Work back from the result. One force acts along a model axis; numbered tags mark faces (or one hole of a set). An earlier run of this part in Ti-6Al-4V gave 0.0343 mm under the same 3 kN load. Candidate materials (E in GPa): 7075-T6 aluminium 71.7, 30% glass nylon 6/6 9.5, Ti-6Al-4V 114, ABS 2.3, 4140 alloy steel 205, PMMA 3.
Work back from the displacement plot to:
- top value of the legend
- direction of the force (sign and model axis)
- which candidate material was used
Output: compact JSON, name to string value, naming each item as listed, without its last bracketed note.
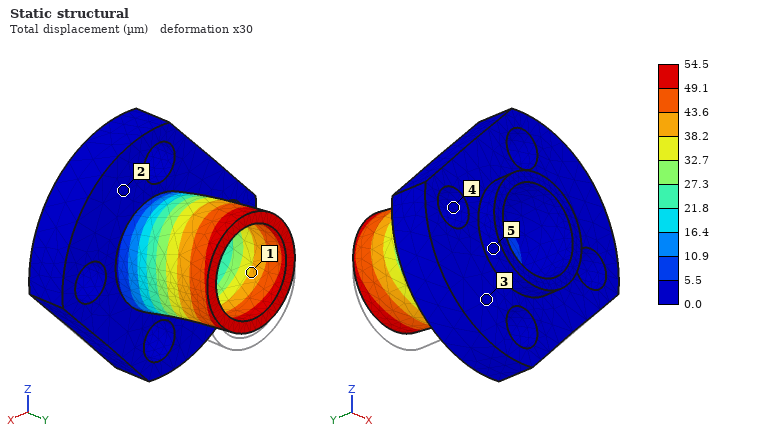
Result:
{"top value of the legend": "54.5 µm", "direction of the force": "+Z", "which candidate material was used": "7075-T6 aluminium"}
